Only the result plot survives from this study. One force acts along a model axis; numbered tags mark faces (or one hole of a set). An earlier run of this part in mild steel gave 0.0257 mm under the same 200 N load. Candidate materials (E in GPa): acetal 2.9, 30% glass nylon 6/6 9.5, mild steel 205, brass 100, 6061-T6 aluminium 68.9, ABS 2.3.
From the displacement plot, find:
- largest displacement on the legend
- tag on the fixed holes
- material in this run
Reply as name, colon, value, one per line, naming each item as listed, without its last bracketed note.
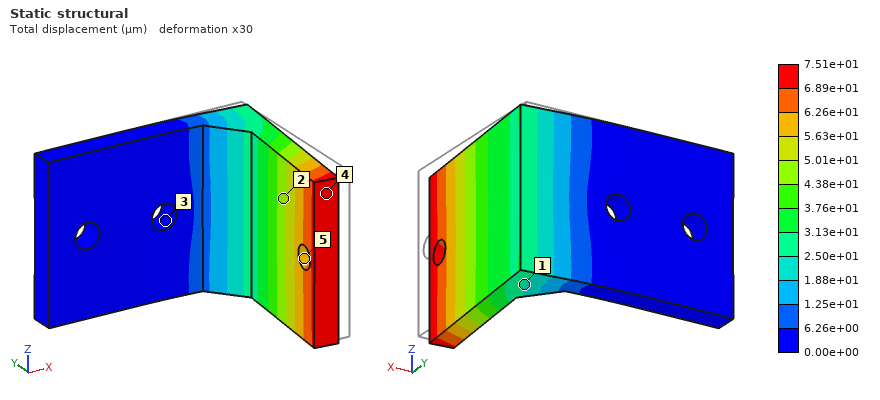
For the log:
largest displacement on the legend: 7.51e+01 µm
tag on the fixed holes: 3
material in this run: 6061-T6 aluminium
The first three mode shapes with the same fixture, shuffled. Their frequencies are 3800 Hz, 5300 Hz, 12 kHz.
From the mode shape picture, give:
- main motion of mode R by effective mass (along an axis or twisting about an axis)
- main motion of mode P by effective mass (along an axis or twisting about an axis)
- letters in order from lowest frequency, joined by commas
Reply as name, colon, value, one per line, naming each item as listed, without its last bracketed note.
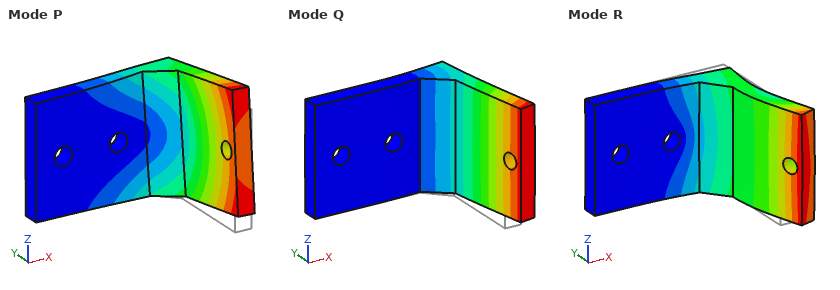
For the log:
main motion of mode R by effective mass: along Y
main motion of mode P by effective mass: along Z
letters in order from lowest frequency, joined by commas: Q, P, R
